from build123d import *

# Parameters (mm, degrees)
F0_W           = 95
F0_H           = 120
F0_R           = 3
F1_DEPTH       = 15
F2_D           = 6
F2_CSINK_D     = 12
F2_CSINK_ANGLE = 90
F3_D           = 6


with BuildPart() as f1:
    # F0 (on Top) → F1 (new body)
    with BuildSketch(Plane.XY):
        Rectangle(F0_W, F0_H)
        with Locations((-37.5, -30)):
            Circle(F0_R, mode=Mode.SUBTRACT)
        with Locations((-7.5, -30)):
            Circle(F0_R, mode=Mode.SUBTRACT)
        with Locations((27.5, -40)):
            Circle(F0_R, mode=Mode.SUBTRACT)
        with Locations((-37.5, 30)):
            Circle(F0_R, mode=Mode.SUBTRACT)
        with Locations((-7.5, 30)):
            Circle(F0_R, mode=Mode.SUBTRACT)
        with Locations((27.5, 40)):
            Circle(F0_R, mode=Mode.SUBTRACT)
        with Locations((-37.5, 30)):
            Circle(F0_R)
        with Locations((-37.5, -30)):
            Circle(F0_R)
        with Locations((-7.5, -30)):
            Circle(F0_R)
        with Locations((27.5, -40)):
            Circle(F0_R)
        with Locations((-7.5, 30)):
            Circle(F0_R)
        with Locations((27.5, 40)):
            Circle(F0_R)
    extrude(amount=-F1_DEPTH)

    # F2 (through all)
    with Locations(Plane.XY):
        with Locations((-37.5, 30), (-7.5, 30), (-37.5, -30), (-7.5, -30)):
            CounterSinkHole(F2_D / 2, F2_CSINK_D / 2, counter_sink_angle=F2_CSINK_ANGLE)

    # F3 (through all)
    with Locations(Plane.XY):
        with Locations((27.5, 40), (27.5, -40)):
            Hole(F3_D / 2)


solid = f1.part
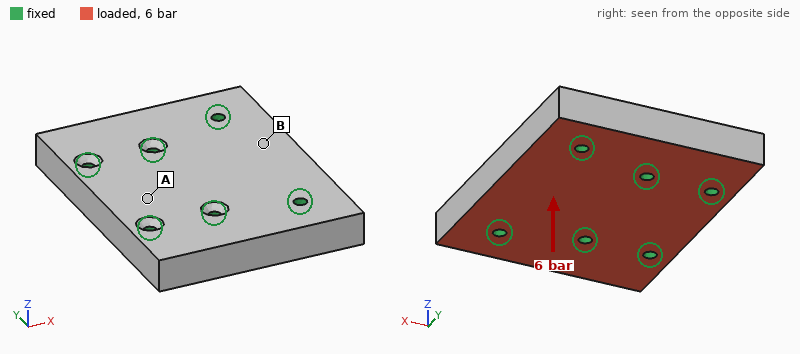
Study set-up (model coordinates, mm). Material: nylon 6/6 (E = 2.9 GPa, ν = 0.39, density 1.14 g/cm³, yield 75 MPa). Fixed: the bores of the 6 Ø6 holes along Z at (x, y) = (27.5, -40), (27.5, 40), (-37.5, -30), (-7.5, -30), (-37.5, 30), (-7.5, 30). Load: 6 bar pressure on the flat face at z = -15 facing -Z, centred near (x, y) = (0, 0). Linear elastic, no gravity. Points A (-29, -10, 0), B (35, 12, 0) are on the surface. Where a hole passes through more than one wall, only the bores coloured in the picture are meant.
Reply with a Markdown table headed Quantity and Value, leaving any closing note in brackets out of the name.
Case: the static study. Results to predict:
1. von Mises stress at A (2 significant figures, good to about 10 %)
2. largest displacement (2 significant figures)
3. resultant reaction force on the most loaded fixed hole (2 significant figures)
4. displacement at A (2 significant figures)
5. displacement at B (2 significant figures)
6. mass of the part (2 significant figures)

| Quantity | Value |
|---|---|
| von Mises stress at A | 1.3 MPa |
| largest displacement | 0.16 mm |
| resultant reaction force on the most loaded fixed hole | 1.4 kN |
| displacement at A | 0.038 mm |
| displacement at B | 0.11 mm |
| mass of the part | 190 g |
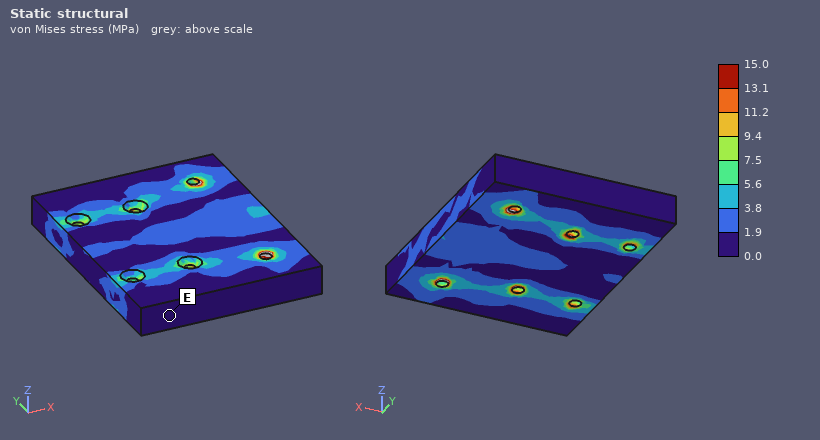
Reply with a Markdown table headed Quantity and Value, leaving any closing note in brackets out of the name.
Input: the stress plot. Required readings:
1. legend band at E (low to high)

| Quantity | Value |
|---|---|
| legend band at E | 0.0 to 1.9 MPa |
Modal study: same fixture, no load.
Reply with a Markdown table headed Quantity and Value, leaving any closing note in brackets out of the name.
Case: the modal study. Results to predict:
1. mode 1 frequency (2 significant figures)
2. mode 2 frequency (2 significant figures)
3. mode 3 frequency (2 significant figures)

| Quantity | Value |
|---|---|
| mode 1 frequency | 2900 Hz |
| mode 2 frequency | 3500 Hz |
| mode 3 frequency | 3500 Hz |
